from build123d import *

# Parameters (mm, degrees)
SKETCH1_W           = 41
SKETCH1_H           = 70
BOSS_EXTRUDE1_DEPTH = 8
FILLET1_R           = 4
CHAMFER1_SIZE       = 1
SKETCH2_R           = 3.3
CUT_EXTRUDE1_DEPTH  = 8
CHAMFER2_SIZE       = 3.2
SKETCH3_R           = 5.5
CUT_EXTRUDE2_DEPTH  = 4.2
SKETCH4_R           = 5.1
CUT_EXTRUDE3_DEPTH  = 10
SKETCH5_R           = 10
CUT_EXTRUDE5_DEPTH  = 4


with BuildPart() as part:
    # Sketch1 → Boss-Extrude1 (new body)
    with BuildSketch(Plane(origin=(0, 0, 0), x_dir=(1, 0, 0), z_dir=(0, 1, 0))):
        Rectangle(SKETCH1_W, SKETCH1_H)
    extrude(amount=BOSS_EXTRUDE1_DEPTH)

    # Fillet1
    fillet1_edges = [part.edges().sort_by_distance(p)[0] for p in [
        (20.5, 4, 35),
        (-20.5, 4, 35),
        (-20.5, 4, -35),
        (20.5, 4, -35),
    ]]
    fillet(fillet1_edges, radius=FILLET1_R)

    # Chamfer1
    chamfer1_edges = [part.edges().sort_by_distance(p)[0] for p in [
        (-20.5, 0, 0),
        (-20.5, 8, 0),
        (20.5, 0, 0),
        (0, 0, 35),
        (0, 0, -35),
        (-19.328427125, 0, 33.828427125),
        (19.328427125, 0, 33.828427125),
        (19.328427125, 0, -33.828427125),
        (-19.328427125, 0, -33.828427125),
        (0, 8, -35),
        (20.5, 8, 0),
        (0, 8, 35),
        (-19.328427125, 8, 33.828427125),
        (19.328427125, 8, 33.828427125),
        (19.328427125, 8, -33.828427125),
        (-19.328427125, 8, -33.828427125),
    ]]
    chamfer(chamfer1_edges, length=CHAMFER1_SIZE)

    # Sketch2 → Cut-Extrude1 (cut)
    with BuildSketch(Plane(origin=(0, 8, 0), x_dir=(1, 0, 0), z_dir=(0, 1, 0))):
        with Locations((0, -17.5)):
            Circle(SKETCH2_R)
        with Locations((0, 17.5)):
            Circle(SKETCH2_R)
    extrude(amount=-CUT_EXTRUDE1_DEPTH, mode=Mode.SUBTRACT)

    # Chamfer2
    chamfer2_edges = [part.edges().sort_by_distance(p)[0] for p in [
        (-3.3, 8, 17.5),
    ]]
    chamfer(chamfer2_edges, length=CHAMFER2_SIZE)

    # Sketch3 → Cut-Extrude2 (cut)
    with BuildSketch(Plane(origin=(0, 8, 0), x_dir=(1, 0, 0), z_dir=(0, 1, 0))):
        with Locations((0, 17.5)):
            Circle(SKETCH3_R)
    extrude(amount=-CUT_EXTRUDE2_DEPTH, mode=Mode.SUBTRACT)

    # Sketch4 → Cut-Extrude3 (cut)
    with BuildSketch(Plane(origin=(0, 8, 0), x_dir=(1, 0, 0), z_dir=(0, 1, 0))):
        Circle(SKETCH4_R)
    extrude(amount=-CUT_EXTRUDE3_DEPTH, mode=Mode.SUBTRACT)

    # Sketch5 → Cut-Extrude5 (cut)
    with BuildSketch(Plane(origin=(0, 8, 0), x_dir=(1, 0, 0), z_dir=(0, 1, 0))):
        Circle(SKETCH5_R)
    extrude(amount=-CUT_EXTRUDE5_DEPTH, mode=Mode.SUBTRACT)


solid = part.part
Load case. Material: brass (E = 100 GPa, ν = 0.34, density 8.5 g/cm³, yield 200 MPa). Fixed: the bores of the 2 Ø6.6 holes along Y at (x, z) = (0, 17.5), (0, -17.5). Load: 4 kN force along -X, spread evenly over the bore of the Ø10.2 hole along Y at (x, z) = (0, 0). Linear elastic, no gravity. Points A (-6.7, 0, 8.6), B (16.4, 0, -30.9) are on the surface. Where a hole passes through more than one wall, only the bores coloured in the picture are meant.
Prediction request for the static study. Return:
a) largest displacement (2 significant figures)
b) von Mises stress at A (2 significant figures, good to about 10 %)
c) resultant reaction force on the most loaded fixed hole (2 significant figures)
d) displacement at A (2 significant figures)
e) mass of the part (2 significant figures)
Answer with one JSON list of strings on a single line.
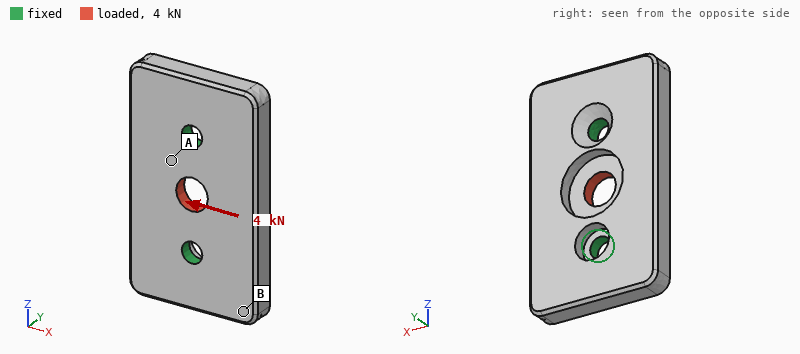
["6.6 µm", "22 MPa", "2.0 kN", "3.3 µm", "170 g"]
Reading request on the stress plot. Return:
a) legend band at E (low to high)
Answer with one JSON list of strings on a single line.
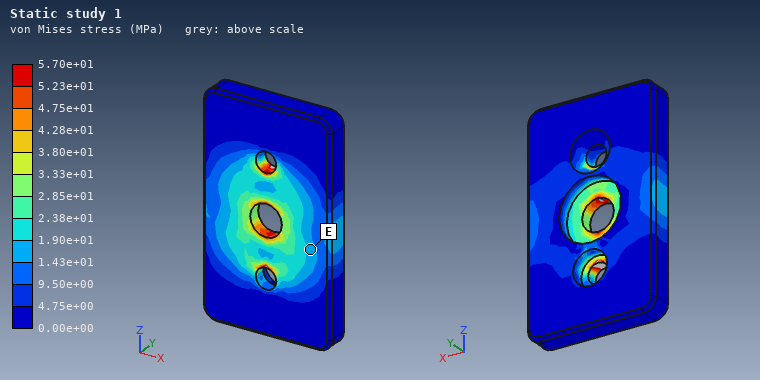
["1.43e+01 to 1.90e+01 MPa"]
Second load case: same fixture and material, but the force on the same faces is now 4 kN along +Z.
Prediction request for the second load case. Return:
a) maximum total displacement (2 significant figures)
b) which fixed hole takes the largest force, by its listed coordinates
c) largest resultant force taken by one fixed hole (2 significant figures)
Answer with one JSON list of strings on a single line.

["4.1 µm", "(0, 17.5)", "2.1 kN"]
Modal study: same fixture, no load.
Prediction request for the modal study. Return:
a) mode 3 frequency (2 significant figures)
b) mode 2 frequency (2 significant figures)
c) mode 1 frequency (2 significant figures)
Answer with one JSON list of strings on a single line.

["7400 Hz", "6900 Hz", "4700 Hz"]
